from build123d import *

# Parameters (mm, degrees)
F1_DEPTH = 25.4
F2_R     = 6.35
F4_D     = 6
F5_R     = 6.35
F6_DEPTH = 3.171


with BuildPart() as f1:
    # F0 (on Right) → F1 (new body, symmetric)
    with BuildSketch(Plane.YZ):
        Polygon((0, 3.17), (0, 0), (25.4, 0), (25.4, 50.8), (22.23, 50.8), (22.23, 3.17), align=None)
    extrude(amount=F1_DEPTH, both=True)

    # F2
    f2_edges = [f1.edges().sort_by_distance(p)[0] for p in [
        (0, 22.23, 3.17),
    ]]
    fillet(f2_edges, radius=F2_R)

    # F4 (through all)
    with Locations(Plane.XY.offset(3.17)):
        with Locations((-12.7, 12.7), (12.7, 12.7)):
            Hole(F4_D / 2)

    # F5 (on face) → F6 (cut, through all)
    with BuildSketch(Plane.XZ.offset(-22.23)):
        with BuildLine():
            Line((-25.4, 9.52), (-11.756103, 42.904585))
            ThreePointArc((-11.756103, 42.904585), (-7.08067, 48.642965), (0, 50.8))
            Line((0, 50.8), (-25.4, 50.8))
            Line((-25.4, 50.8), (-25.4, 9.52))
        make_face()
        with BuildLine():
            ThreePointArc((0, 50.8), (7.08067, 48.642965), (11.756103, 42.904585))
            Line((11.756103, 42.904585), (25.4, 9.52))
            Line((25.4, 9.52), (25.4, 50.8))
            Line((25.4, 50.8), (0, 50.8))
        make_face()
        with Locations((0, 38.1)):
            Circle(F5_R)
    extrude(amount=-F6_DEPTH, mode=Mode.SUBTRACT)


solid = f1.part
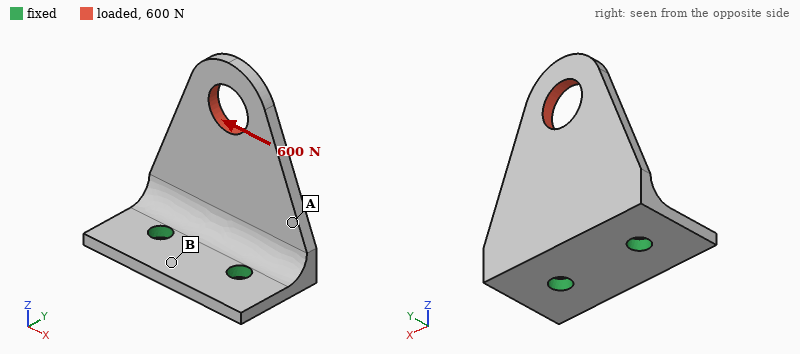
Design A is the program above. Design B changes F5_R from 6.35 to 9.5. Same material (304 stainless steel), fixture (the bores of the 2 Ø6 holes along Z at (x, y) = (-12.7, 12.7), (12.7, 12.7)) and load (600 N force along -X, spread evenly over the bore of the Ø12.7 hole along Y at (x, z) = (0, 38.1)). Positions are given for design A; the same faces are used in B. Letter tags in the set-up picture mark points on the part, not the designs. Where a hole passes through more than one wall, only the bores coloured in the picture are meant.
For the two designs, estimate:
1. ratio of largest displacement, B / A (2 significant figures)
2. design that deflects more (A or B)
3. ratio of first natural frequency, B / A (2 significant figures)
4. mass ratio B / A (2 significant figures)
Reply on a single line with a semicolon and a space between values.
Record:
1.2; B; 1.2; 0.95
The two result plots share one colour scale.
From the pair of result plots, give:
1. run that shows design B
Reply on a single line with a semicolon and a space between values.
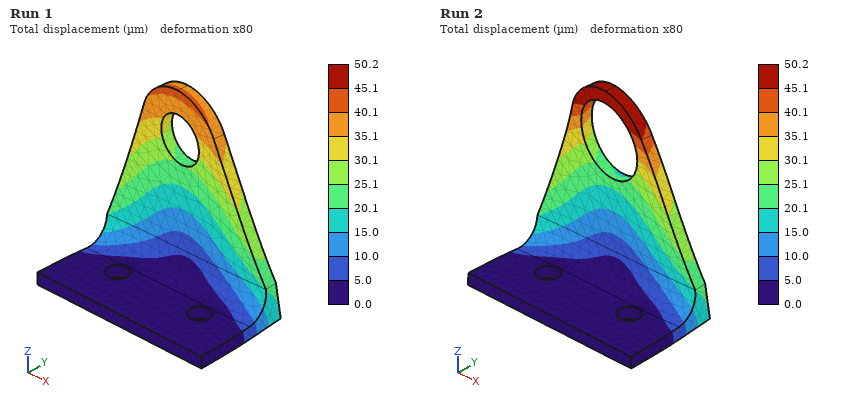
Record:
Run 2
